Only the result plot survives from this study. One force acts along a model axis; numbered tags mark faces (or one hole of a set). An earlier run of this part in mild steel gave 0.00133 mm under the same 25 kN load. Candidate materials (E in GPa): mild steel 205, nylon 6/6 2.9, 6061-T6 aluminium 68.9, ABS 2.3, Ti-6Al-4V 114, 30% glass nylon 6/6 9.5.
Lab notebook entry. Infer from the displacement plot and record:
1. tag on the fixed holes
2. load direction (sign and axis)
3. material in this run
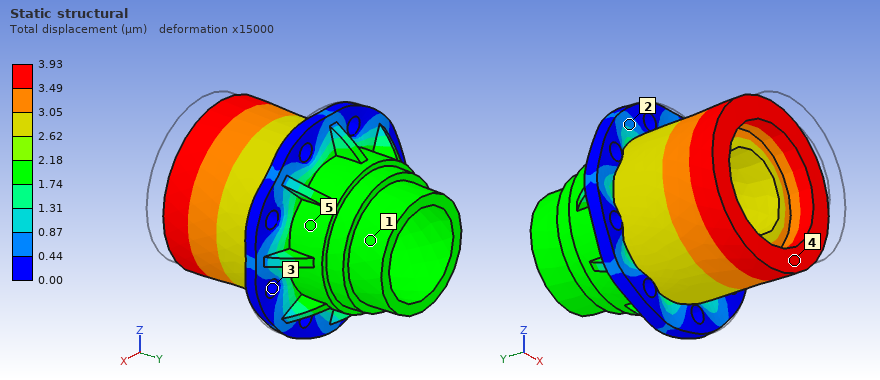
3
+Y
6061-T6 aluminium
